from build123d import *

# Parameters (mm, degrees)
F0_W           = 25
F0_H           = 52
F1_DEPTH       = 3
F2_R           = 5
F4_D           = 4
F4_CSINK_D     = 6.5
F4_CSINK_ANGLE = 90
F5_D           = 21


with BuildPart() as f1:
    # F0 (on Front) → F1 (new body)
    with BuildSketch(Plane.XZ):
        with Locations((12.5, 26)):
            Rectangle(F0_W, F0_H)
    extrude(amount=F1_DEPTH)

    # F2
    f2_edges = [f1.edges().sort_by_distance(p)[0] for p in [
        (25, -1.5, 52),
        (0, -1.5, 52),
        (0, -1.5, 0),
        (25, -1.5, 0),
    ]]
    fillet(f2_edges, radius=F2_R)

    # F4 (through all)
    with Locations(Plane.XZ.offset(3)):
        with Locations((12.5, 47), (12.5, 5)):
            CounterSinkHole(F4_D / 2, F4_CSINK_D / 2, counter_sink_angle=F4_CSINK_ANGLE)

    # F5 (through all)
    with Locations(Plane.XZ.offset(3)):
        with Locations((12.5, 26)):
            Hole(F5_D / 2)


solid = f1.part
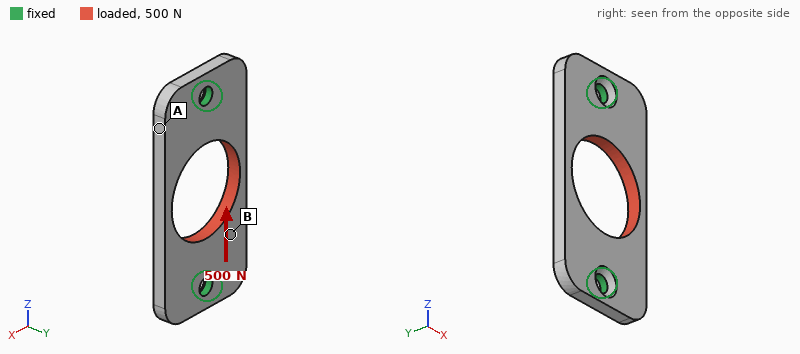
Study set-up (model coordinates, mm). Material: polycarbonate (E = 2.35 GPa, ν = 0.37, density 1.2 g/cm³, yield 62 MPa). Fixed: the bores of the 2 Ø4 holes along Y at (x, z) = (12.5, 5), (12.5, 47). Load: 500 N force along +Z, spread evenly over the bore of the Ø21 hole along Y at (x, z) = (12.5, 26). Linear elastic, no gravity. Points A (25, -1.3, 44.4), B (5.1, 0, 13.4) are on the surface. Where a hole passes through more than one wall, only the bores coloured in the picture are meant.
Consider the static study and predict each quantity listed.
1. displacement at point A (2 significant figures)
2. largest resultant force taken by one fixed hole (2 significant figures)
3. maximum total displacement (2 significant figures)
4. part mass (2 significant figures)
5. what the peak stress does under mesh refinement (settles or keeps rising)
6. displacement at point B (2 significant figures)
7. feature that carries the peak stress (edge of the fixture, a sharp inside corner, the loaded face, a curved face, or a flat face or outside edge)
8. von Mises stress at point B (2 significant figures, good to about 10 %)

47 µm
250 N
77 µm
3.2 g
keeps rising
43 µm
edge of the fixture
5.7 MPa
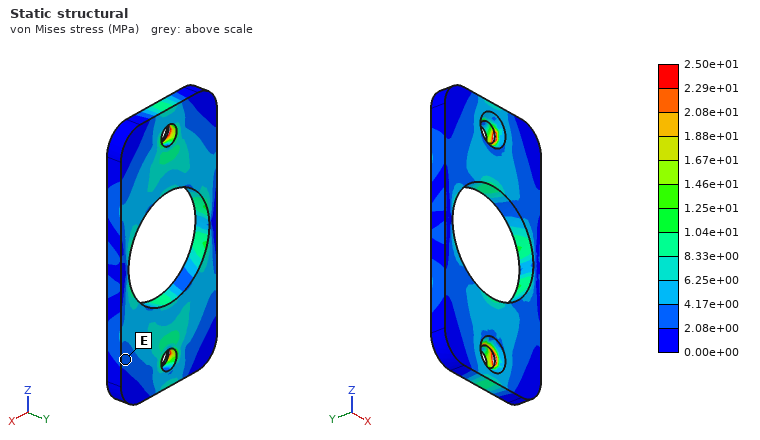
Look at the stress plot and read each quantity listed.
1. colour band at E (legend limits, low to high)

2.08e+00 to 4.17e+00 MPa
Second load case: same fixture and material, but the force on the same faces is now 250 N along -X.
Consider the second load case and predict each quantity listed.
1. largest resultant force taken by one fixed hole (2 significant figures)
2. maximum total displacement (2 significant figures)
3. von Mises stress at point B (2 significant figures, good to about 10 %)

130 N
0.12 mm
3.4 MPa
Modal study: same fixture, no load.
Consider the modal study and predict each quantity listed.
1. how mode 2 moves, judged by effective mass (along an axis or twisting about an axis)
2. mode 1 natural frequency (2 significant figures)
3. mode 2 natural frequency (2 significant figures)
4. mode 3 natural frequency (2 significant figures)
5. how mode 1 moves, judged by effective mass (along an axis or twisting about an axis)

along Y
2100 Hz
2300 Hz
3400 Hz
twisting about Z
